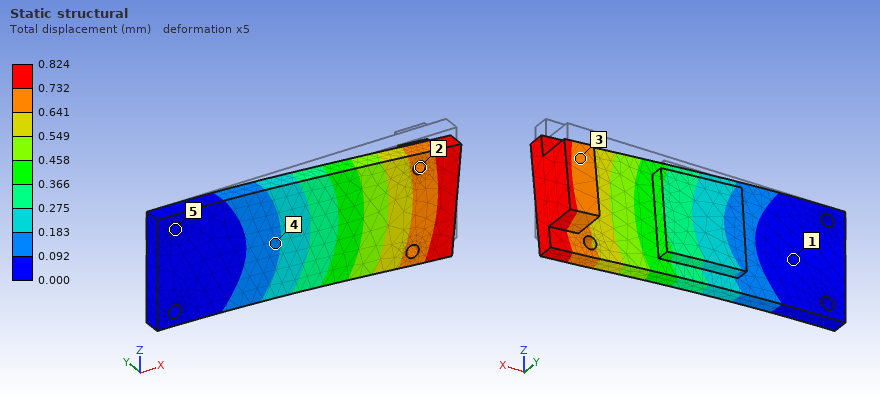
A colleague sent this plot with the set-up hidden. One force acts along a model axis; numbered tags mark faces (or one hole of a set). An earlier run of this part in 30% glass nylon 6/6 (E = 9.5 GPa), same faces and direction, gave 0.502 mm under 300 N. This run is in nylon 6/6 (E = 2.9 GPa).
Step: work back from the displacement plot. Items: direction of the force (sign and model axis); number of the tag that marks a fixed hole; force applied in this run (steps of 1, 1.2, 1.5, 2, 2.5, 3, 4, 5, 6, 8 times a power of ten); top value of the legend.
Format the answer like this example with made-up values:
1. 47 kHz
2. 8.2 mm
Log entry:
1. -Z
2. 5
3. 150 N
4. 0.824 mm
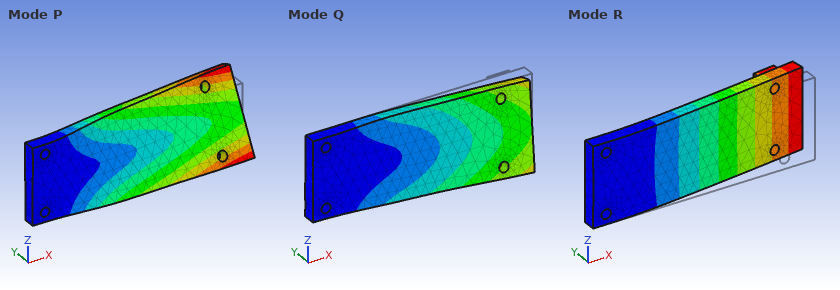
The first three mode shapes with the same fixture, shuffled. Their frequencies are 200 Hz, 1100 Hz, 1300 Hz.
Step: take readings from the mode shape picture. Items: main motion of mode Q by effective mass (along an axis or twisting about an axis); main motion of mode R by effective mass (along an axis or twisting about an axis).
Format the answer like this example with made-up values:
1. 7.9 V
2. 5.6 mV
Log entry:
1. along Z
2. along Y
